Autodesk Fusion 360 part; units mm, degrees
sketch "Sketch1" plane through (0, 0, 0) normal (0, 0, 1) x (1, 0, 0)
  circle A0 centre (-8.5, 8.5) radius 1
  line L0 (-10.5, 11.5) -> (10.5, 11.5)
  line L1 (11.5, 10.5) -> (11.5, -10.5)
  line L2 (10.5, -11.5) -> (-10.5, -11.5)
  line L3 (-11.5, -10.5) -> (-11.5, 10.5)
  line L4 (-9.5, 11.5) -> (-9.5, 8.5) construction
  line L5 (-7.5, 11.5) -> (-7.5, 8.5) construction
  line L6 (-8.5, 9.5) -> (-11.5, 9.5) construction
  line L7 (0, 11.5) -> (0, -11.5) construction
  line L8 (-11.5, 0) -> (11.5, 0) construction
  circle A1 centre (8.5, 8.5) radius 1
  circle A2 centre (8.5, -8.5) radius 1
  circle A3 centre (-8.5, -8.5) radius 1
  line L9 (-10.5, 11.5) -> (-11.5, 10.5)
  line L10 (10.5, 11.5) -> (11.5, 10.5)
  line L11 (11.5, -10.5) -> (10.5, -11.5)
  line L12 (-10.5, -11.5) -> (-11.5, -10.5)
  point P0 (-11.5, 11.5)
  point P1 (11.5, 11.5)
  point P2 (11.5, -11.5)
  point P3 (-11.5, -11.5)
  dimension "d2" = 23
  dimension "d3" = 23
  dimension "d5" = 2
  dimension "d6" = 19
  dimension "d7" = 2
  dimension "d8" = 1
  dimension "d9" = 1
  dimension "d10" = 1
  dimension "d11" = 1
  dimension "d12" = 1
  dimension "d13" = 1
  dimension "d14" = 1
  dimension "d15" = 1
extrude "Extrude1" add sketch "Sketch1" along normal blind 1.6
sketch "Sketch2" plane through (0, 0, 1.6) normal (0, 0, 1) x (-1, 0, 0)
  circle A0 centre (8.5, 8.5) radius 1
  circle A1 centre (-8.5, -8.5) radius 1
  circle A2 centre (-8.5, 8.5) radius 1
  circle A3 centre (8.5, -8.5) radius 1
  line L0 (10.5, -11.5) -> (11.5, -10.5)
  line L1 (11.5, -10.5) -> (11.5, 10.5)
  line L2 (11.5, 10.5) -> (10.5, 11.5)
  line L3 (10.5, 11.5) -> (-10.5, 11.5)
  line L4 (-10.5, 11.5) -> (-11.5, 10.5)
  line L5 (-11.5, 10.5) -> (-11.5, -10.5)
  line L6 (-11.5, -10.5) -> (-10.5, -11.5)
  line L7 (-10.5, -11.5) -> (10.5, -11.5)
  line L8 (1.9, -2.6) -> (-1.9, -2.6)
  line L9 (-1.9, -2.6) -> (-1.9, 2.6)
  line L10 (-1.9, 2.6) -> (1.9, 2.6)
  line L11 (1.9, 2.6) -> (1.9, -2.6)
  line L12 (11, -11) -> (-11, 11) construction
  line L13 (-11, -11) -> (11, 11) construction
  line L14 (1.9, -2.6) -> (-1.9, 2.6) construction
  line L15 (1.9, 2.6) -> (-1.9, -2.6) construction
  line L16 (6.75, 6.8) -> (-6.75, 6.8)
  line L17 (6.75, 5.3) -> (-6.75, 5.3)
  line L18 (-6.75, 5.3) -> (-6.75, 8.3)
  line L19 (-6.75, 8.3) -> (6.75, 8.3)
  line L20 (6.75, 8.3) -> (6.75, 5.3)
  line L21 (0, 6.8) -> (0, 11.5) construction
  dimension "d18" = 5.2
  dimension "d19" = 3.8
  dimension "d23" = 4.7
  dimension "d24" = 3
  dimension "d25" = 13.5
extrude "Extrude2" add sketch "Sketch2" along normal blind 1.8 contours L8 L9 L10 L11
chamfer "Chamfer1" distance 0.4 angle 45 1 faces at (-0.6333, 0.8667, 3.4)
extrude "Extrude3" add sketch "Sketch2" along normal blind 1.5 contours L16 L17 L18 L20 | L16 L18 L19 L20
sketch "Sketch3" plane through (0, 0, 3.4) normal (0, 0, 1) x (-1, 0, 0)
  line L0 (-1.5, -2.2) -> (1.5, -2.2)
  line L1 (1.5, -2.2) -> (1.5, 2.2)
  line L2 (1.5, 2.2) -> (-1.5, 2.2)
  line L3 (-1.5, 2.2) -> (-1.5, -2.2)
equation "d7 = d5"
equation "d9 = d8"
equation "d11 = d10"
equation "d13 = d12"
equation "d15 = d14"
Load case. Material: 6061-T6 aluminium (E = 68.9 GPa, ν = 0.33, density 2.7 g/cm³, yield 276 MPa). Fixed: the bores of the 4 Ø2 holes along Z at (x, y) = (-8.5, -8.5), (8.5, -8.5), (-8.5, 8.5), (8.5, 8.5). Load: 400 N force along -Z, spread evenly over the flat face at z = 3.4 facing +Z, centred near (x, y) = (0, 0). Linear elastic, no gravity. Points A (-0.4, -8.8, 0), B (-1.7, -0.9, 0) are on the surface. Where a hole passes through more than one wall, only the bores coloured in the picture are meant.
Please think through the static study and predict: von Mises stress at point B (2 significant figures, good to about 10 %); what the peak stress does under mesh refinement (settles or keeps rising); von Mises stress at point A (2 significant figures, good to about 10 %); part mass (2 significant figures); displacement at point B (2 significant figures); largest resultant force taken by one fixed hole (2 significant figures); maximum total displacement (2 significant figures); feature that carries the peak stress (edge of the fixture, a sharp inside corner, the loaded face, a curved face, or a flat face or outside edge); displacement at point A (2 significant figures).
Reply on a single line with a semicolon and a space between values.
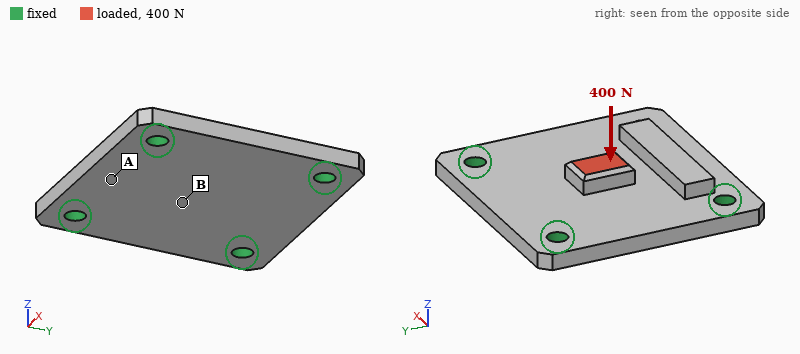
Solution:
86 MPa; keeps rising; 27 MPa; 2.5 g; 35 µm; 120 N; 37 µm; edge of the fixture; 7.3 µm
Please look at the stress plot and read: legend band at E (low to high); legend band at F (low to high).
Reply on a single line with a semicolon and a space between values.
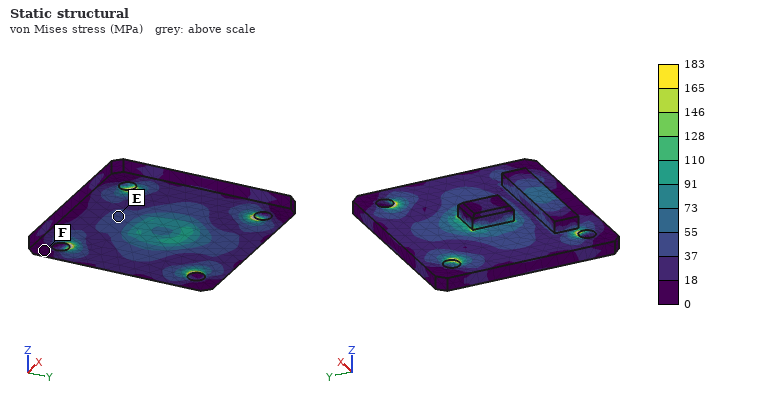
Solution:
37 to 55 MPa; 0 to 18 MPa
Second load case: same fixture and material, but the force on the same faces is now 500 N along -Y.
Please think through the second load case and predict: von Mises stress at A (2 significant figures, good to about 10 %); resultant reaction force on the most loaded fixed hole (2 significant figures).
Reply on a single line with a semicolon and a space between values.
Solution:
18 MPa; 160 N
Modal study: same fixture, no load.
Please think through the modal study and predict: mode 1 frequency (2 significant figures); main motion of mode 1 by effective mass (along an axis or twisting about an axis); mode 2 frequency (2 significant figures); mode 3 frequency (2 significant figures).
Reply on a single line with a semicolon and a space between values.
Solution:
21 kHz; along Z; 33 kHz; 33 kHz
